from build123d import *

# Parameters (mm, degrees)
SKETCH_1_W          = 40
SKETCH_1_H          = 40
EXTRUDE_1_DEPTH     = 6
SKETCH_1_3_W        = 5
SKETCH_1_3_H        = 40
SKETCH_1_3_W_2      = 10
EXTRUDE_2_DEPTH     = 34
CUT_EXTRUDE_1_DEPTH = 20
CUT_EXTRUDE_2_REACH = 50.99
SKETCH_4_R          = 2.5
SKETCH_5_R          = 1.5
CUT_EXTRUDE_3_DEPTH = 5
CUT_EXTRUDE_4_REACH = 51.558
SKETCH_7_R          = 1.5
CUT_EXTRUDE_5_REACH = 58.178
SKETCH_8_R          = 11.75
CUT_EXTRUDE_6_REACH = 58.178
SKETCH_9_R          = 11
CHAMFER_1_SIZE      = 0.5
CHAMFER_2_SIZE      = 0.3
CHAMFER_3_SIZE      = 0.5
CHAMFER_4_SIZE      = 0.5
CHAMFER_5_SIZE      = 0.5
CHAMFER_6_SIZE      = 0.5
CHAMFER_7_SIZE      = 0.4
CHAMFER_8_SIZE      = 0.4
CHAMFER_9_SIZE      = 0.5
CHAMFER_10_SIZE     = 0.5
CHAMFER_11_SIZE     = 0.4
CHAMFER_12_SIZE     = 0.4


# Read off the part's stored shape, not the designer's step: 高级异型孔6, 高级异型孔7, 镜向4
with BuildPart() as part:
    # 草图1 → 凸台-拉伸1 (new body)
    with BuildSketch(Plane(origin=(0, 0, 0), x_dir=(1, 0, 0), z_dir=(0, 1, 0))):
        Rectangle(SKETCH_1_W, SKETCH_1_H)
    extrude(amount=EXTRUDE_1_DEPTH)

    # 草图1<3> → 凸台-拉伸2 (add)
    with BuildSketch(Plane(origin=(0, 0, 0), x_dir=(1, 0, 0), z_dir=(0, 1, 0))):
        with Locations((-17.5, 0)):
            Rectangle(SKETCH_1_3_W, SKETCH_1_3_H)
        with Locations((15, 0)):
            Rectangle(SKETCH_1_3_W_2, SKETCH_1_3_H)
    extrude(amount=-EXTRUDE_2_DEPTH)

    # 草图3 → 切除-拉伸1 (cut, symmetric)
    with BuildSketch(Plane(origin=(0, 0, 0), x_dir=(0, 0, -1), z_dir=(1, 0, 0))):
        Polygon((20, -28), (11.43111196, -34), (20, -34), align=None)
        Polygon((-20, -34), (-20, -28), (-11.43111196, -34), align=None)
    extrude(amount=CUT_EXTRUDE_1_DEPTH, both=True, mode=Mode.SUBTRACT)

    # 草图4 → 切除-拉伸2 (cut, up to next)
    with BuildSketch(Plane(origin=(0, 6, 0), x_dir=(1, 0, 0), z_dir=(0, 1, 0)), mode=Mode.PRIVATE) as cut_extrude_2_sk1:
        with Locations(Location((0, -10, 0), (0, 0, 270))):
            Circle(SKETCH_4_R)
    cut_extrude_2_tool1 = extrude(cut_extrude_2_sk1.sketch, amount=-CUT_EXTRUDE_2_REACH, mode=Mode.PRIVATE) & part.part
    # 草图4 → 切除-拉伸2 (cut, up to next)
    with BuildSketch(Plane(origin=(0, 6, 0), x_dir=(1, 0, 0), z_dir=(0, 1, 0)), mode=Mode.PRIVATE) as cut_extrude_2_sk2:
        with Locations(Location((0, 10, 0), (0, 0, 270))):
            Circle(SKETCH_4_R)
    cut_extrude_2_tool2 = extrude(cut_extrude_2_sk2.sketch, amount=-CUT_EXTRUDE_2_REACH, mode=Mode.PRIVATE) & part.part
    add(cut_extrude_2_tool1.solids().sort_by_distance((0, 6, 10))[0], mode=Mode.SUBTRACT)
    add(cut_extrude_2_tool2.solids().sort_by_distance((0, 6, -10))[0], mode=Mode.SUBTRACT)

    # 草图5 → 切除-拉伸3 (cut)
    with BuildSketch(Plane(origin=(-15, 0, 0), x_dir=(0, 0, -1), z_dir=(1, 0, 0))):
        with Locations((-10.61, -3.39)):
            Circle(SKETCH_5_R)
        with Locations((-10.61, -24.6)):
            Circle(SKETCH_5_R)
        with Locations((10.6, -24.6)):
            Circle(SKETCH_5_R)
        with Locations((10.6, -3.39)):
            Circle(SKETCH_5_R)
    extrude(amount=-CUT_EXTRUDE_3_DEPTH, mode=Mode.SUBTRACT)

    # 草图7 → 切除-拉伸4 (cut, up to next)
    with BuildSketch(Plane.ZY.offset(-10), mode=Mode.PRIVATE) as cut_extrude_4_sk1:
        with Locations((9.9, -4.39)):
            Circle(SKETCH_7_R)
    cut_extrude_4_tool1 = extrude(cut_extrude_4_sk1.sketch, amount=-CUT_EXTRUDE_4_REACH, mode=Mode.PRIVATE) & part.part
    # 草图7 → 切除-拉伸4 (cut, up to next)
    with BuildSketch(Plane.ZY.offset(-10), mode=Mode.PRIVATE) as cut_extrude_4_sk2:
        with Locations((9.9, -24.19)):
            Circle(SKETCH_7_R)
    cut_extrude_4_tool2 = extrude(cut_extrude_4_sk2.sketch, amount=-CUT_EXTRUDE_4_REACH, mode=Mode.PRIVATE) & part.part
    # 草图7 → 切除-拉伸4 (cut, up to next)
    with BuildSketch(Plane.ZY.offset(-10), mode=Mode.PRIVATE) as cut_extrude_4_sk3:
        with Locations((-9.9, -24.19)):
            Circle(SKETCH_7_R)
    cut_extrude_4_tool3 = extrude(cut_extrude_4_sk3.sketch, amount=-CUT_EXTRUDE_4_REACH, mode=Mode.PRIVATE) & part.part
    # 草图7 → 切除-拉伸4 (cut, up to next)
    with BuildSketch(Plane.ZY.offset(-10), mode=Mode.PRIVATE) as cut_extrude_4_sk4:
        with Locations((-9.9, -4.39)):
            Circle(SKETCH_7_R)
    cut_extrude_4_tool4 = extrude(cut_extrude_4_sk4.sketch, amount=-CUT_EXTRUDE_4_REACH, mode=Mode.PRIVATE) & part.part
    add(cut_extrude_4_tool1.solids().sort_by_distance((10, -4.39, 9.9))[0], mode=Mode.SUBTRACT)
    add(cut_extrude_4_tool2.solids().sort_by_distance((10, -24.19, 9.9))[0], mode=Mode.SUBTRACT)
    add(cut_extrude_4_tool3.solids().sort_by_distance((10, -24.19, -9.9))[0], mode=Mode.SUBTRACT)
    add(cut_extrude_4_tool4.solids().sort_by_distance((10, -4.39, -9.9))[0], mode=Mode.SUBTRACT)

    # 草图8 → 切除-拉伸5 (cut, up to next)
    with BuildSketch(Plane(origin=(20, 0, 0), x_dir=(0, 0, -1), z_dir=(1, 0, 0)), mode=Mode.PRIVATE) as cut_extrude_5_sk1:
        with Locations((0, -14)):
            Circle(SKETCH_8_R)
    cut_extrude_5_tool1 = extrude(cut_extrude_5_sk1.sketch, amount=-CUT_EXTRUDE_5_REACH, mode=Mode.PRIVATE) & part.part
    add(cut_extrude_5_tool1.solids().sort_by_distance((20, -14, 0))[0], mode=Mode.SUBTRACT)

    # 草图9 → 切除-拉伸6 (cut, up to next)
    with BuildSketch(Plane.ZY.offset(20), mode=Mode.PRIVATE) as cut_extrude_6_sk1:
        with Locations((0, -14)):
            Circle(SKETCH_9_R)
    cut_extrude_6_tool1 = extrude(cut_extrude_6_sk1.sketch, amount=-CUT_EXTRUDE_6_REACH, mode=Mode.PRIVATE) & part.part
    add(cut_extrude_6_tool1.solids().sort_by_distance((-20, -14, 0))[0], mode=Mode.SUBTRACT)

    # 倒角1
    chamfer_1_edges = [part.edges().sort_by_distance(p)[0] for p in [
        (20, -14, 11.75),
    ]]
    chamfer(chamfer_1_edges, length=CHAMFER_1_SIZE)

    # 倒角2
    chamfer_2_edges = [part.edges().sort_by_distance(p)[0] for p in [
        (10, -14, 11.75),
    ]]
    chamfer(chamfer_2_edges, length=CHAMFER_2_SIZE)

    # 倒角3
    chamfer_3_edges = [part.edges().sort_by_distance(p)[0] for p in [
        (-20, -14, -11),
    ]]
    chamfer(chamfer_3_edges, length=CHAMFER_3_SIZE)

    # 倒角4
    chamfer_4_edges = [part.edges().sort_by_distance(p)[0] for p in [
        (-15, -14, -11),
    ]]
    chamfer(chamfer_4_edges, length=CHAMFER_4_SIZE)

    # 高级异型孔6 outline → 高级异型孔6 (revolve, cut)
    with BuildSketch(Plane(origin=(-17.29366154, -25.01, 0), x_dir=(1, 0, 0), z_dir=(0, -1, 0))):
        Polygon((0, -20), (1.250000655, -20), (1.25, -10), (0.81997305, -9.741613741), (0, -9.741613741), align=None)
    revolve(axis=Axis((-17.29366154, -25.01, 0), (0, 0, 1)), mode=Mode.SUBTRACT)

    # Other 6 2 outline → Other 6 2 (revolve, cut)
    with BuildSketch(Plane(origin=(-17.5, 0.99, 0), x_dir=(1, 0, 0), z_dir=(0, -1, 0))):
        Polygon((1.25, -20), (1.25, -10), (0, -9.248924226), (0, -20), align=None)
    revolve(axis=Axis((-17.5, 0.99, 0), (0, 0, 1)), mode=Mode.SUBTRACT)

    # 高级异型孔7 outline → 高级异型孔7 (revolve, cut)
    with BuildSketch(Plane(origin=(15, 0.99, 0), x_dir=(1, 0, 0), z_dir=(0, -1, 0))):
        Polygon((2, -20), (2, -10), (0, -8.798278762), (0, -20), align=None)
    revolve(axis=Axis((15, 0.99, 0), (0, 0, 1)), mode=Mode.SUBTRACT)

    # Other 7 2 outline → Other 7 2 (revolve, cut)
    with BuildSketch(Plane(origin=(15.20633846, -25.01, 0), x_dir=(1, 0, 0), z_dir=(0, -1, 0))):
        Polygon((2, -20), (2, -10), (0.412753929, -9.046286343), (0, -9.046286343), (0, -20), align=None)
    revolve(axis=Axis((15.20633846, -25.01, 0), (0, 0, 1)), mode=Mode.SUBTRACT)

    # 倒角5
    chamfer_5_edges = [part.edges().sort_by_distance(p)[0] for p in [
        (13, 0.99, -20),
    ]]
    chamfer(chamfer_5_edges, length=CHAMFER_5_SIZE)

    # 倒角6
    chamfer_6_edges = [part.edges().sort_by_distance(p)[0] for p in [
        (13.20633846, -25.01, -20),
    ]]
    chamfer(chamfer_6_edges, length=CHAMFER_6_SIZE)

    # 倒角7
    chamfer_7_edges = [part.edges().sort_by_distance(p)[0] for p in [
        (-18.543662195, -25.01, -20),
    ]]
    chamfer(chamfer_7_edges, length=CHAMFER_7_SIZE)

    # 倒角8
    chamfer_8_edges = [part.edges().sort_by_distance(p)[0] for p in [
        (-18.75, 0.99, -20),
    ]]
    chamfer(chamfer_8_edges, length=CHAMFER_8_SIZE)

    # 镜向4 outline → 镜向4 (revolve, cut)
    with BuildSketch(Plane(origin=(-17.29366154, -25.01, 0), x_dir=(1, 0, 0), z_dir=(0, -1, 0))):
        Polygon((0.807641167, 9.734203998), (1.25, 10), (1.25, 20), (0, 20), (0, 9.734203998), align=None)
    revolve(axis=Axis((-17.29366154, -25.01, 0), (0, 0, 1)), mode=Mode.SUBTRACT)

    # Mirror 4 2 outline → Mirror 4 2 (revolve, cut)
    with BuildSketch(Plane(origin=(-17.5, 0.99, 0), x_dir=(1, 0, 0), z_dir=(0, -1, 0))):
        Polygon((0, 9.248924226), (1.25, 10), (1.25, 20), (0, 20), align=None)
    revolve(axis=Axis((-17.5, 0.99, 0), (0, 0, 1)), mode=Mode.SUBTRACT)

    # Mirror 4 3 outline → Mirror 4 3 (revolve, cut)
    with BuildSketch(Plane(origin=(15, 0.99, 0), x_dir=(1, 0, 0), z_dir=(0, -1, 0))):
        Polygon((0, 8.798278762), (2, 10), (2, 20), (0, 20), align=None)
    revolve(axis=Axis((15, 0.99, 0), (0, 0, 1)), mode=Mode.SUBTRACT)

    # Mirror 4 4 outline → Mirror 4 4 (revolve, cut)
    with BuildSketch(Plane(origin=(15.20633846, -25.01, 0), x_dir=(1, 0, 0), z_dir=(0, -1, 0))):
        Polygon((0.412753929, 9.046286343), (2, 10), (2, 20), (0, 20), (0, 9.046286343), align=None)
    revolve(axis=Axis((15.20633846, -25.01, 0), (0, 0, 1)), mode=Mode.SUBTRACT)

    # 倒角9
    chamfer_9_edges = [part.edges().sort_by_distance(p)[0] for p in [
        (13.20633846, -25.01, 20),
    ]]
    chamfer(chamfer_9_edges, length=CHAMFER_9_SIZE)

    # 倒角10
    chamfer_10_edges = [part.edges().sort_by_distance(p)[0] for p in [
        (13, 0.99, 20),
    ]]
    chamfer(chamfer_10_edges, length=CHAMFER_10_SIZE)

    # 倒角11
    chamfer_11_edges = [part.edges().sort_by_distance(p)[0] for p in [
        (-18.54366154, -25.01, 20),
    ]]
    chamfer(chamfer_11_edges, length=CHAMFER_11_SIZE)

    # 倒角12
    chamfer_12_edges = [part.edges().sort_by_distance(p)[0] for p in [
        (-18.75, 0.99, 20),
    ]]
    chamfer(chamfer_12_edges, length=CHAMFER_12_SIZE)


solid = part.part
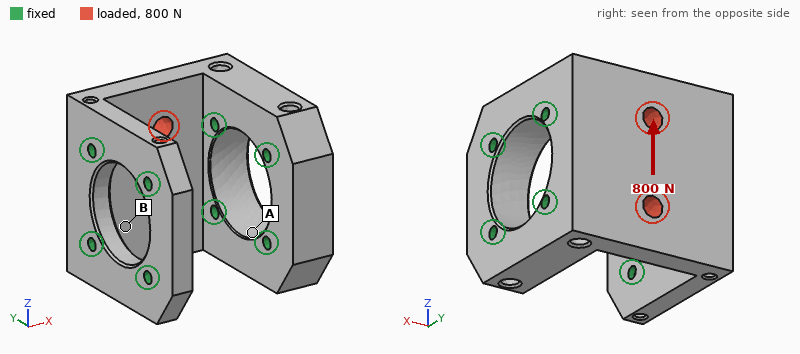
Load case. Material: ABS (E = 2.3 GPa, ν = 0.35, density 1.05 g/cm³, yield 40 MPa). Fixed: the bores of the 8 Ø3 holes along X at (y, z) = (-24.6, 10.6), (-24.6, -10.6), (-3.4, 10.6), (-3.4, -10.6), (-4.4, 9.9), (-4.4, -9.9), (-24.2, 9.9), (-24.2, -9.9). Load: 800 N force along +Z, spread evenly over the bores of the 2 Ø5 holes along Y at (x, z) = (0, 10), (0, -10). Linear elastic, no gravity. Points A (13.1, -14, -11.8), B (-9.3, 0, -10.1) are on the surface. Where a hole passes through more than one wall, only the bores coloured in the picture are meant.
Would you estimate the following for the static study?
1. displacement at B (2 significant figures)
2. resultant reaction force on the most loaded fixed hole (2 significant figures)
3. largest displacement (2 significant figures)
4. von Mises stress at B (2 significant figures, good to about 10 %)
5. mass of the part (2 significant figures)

33 µm
260 N
58 µm
2.8 MPa
23 g
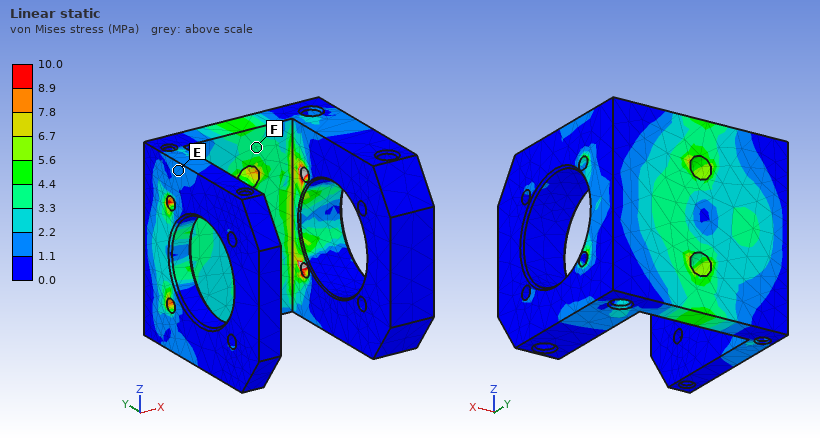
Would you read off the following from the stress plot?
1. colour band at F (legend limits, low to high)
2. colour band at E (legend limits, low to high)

3.3 to 4.4 MPa
1.1 to 2.2 MPa
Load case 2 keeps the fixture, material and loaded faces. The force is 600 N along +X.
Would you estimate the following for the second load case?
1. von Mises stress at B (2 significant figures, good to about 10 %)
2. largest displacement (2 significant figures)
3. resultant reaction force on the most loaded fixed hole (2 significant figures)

3.2 MPa
38 µm
190 N
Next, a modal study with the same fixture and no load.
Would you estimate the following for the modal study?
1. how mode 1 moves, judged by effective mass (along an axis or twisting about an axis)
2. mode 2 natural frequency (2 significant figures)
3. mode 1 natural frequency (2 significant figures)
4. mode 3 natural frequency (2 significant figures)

along Y
7400 Hz
6700 Hz
7600 Hz
